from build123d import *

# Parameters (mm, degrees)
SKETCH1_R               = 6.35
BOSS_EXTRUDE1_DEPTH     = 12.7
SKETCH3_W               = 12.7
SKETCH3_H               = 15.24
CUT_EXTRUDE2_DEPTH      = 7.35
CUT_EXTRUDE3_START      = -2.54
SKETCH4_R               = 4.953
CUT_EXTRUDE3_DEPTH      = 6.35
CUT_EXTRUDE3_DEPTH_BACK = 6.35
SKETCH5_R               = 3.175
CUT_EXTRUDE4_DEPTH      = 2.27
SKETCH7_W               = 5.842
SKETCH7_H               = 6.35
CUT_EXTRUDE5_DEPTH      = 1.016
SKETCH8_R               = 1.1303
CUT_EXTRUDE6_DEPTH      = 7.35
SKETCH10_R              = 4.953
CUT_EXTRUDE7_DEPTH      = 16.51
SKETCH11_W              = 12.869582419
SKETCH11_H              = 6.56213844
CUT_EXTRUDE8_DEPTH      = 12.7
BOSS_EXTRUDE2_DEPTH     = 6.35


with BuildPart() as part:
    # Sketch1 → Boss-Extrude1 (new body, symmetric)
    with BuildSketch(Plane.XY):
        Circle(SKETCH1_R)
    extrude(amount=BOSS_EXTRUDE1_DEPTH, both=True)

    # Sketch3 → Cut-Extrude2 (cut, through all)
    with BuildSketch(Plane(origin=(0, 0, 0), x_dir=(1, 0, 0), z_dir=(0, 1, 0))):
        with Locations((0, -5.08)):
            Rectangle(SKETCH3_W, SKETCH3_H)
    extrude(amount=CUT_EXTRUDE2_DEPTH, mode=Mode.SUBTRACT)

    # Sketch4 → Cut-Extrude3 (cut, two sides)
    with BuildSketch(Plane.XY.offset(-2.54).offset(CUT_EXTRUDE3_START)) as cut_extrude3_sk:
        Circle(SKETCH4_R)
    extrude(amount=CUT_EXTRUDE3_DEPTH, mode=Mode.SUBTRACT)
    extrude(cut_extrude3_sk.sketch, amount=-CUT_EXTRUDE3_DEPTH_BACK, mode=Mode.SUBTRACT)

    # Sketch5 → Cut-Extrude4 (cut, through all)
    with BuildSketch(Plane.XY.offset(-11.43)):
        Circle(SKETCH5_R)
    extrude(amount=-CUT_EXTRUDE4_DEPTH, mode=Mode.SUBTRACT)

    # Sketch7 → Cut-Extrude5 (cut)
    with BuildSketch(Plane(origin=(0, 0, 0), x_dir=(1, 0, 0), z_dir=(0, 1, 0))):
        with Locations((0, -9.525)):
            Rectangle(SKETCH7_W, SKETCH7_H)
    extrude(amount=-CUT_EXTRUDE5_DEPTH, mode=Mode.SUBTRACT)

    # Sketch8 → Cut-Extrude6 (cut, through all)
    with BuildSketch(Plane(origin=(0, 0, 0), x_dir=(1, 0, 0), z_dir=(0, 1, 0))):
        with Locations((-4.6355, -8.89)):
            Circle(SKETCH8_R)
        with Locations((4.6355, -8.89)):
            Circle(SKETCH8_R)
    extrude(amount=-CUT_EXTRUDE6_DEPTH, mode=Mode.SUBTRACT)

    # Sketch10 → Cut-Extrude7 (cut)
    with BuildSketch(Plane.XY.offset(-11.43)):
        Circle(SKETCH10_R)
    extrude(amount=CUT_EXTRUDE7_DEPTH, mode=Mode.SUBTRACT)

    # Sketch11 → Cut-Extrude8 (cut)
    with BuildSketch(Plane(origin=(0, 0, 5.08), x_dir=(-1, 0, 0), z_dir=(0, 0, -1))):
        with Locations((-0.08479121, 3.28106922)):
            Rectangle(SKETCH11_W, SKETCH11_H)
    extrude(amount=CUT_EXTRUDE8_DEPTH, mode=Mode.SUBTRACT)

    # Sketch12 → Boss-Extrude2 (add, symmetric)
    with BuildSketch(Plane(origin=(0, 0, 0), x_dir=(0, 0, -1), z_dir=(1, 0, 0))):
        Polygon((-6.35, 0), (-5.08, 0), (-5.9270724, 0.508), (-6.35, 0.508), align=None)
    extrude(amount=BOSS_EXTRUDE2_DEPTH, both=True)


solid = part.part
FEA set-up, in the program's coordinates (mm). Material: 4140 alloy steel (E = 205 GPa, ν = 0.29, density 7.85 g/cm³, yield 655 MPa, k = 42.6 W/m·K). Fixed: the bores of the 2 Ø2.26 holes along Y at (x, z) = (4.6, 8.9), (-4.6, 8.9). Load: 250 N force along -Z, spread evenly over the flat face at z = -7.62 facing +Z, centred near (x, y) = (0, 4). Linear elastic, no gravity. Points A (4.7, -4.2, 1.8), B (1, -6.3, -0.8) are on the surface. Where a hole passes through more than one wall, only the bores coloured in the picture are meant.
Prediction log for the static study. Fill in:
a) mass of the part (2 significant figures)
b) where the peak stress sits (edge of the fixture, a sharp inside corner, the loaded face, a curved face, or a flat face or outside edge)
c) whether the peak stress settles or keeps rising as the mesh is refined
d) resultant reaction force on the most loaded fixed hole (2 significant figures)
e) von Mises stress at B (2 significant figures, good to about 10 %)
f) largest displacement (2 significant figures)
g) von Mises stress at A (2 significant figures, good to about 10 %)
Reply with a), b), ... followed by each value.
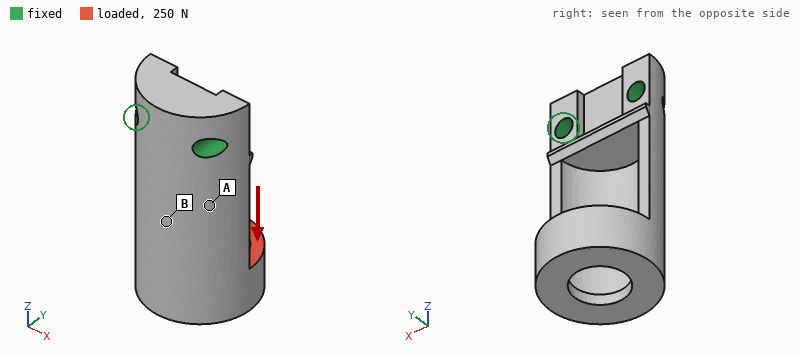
a) 8.2 g
b) a sharp inside corner
c) keeps rising
d) 140 N
e) 55 MPa
f) 41 µm
g) 15 MPa
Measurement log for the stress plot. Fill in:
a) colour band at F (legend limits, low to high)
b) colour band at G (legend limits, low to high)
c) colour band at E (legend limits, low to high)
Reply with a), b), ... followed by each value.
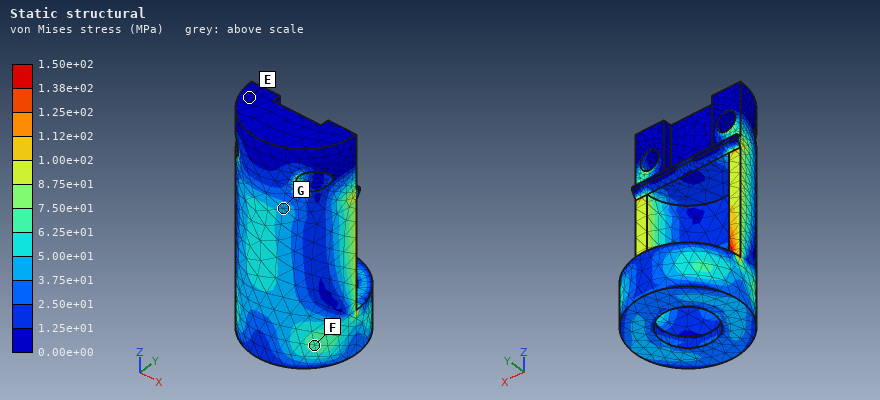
a) 6.25e+01 to 7.50e+01 MPa
b) 3.75e+01 to 5.00e+01 MPa
c) 0.00e+00 to 1.25e+01 MPa
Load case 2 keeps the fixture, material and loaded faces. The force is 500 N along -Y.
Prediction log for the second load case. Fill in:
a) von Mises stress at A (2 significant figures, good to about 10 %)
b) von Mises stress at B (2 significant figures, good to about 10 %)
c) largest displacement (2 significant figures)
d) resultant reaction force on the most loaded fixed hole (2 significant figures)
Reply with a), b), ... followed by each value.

a) 100 MPa
b) 110 MPa
c) 73 µm
d) 290 N
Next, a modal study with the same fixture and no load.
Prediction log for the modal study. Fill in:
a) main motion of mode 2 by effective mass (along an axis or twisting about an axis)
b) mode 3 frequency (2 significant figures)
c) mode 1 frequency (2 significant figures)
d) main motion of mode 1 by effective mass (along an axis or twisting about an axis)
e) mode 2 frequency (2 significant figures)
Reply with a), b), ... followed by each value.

a) along Y
b) 19 kHz
c) 5000 Hz
d) along X
e) 7000 Hz
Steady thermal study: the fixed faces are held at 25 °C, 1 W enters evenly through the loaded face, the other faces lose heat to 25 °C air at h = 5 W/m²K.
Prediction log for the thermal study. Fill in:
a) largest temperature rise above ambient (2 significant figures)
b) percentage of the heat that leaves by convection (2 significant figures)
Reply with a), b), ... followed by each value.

a) 25 K
b) 6.3 %
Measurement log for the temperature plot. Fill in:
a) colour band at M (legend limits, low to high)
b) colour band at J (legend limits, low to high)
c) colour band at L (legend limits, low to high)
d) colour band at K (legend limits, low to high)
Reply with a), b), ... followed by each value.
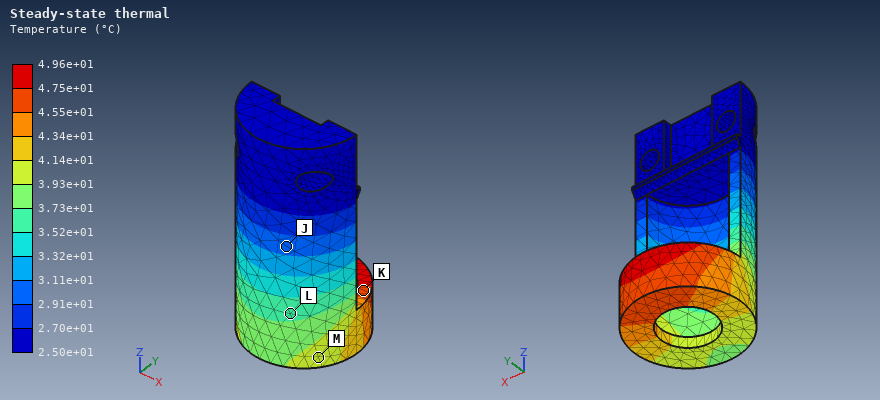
a) 3.93e+01 to 4.14e+01 °C
b) 2.91e+01 to 3.11e+01 °C
c) 3.52e+01 to 3.73e+01 °C
d) 4.55e+01 to 4.75e+01 °C
